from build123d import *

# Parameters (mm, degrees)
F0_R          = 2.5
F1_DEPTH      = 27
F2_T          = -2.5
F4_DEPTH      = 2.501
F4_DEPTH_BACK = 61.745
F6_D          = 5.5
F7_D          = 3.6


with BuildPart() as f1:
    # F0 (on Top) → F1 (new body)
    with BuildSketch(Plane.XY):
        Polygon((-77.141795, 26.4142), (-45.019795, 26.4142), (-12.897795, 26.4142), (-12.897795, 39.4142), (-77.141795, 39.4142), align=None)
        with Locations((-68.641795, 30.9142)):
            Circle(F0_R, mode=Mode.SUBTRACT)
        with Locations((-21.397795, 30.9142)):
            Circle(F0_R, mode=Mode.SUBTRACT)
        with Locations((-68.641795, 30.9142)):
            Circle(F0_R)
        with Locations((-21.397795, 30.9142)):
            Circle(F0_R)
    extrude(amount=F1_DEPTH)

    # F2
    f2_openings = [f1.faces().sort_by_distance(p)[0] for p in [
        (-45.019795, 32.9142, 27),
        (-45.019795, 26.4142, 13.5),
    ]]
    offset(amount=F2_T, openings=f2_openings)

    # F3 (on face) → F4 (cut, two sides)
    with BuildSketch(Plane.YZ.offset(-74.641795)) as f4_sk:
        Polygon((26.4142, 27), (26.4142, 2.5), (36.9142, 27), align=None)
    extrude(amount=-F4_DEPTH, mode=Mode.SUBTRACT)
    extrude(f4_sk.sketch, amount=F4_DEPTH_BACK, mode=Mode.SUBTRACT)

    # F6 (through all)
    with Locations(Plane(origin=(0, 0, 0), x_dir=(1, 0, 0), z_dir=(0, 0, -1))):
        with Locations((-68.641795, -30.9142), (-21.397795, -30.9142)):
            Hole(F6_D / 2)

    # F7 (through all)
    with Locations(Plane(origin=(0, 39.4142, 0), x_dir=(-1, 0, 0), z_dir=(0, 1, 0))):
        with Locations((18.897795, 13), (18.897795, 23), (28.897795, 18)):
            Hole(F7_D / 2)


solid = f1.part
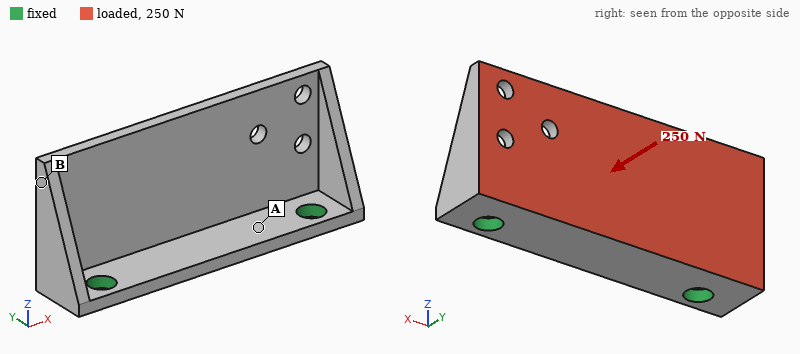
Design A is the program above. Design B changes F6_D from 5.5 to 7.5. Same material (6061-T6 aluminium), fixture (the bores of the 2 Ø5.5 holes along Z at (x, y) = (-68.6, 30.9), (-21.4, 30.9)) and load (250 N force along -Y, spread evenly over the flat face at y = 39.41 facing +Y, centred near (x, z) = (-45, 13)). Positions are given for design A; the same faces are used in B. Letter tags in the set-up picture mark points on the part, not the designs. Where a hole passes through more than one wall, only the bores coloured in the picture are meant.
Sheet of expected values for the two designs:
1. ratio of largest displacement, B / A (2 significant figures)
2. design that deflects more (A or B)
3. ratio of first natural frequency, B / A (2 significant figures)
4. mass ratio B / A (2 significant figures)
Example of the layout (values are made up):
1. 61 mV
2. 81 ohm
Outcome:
1. 0.83
2. A
3. 1.1
4. 0.98
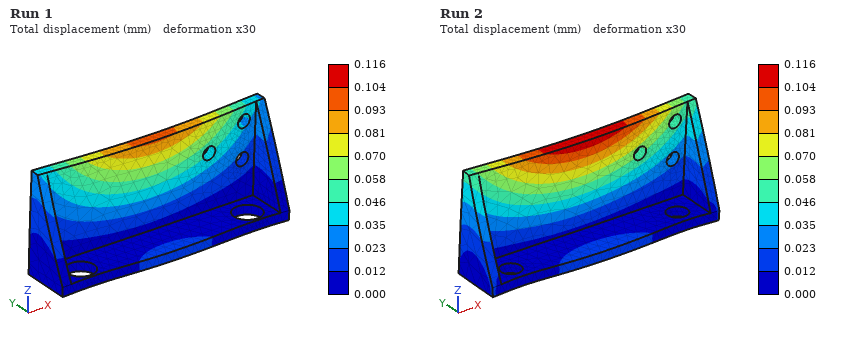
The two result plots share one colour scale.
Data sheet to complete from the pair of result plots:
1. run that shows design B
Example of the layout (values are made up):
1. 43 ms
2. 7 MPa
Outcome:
1. Run 1
